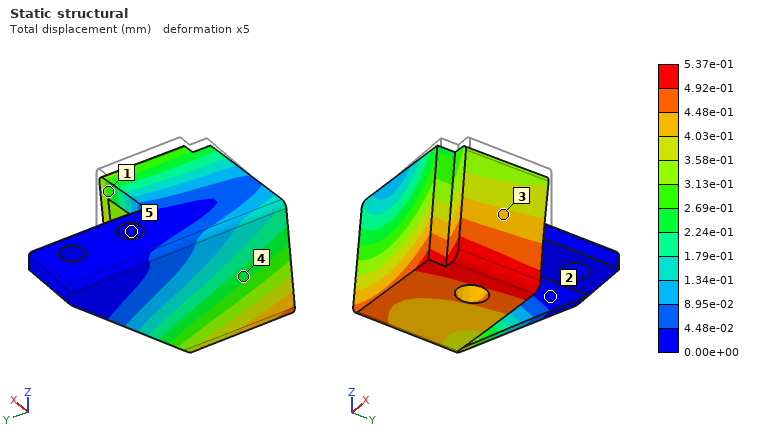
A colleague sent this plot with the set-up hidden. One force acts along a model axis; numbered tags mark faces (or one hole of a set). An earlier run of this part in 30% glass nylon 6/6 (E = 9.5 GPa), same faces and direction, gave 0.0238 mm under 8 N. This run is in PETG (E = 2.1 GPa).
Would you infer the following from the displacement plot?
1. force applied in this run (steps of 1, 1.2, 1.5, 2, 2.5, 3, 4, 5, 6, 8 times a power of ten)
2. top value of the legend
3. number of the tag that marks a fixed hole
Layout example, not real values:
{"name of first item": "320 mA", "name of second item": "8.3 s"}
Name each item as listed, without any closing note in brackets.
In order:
{"force applied in this run": "40 N", "top value of the legend": "5.37e-01 mm", "number of the tag that marks a fixed hole": "5"}
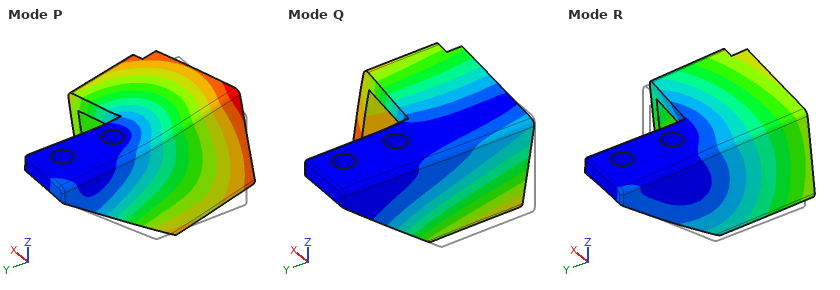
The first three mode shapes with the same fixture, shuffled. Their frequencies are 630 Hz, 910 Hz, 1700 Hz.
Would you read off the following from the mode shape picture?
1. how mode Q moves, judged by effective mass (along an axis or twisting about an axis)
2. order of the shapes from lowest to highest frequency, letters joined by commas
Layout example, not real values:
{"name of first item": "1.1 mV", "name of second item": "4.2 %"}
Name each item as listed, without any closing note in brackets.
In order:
{"how mode Q moves, judged by effective mass": "along X", "order of the shapes from lowest to highest frequency, letters joined by commas": "Q, R, P"}
